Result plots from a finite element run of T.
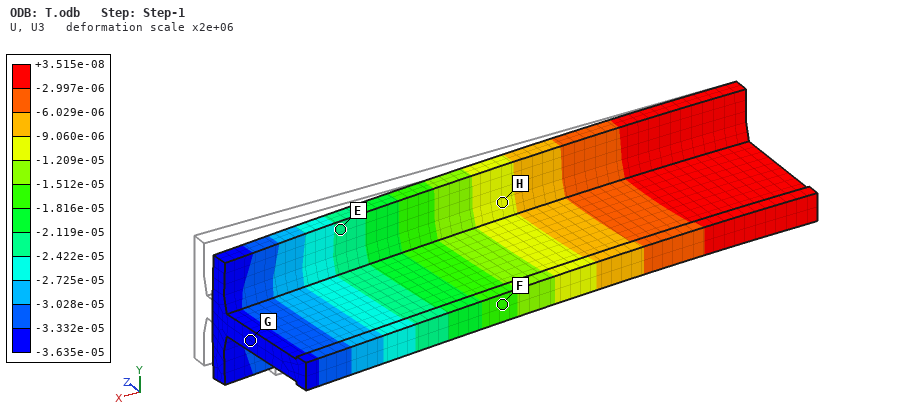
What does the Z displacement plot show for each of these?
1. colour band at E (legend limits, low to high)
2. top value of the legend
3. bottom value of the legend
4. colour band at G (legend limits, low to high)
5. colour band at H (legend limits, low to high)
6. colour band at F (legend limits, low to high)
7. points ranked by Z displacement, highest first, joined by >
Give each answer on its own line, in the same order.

-2.422e-05 to -2.119e-05
+3.515e-08
-3.635e-05
-3.635e-05 to -3.332e-05
-1.209e-05 to -9.060e-06
-1.816e-05 to -1.512e-05
H > F > E > G
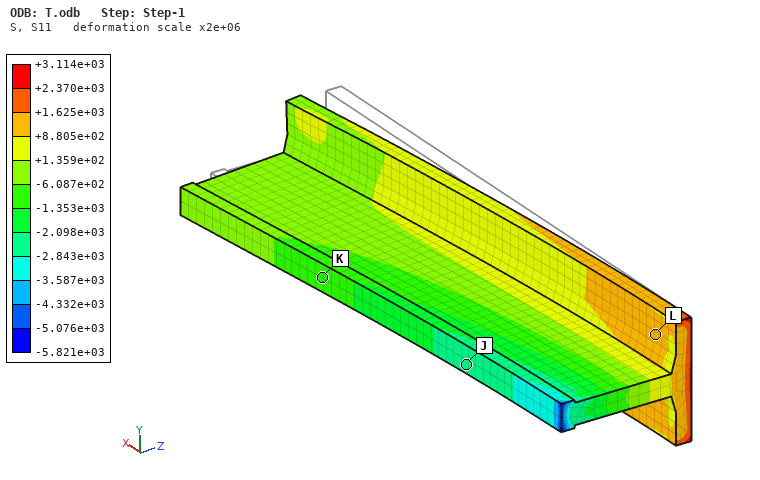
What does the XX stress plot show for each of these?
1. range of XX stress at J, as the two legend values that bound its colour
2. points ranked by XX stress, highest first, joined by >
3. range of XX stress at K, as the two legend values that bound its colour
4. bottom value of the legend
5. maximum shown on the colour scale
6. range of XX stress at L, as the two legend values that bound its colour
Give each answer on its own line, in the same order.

-2.843e+03 to -2.098e+03
L > K > J
-1.353e+03 to -6.087e+02
-5.821e+03
+3.114e+03
+8.805e+02 to +1.625e+03
